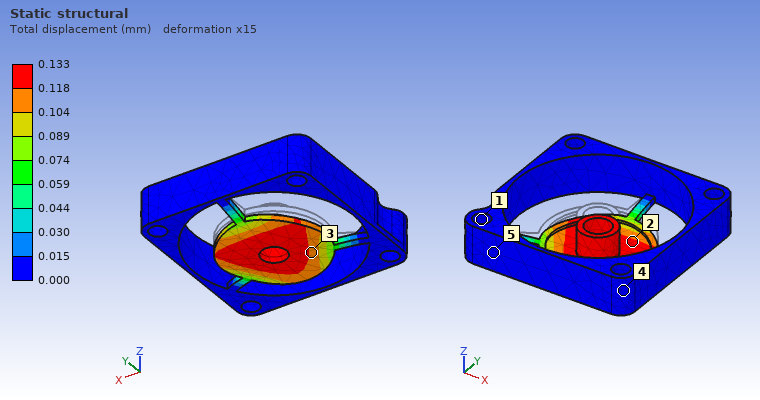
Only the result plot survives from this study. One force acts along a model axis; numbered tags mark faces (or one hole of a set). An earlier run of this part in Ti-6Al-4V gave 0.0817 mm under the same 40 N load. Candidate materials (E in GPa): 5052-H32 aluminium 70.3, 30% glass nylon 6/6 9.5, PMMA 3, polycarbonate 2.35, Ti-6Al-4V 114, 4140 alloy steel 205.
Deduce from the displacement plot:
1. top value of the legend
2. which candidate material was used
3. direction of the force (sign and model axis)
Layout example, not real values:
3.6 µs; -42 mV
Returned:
0.133 mm; 5052-H32 aluminium; -Z
